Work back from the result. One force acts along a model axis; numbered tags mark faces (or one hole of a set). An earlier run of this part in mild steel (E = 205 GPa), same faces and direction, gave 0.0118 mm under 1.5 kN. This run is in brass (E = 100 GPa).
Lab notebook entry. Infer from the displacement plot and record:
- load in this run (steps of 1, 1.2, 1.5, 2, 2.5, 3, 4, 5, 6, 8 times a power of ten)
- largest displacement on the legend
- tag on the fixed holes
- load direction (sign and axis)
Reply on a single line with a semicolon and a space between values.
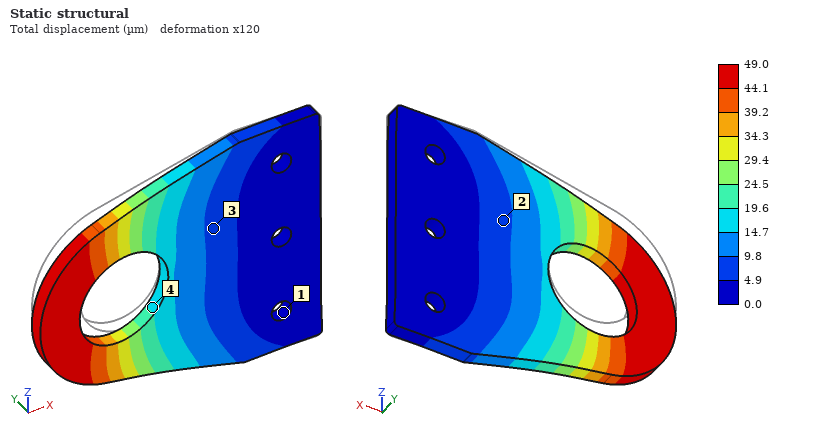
3 kN; 49.0 µm; 1; -Z
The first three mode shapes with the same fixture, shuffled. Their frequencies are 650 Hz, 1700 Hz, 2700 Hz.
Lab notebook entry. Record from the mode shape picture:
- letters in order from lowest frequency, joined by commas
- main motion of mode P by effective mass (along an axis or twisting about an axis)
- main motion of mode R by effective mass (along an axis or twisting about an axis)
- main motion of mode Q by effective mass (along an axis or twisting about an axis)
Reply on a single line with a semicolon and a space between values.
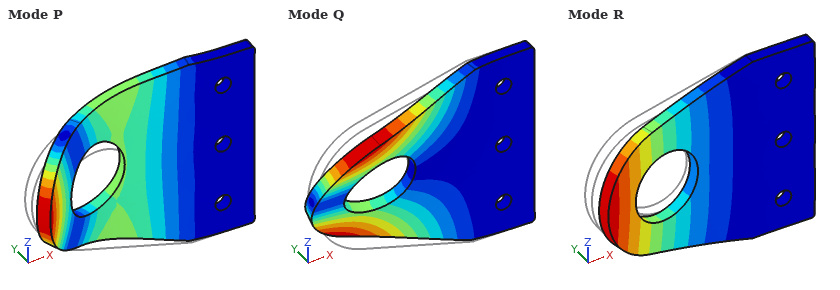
R, Q, P; along Y; along Y; twisting about X
